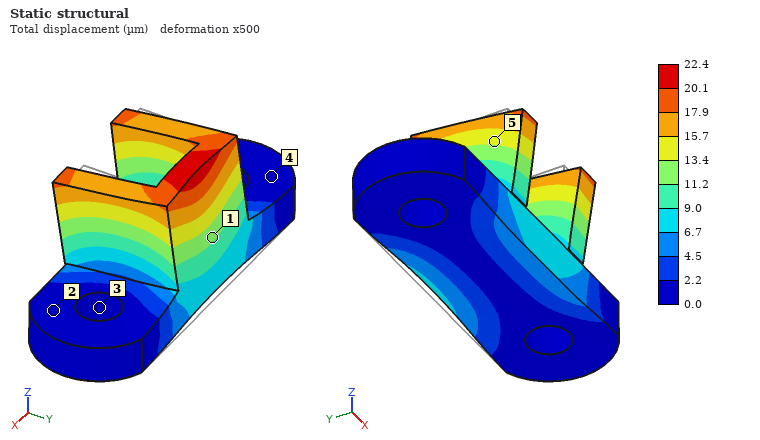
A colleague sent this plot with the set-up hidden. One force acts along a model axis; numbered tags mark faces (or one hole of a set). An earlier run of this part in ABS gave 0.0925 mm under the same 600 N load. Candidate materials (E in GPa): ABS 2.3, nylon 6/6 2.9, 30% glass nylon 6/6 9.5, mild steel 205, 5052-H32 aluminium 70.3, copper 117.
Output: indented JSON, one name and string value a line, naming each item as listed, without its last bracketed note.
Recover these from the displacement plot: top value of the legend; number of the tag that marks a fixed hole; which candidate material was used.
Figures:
{
  "top value of the legend": "22.4 µm",
  "number of the tag that marks a fixed hole": "3",
  "which candidate material was used": "30% glass nylon 6/6"
}
